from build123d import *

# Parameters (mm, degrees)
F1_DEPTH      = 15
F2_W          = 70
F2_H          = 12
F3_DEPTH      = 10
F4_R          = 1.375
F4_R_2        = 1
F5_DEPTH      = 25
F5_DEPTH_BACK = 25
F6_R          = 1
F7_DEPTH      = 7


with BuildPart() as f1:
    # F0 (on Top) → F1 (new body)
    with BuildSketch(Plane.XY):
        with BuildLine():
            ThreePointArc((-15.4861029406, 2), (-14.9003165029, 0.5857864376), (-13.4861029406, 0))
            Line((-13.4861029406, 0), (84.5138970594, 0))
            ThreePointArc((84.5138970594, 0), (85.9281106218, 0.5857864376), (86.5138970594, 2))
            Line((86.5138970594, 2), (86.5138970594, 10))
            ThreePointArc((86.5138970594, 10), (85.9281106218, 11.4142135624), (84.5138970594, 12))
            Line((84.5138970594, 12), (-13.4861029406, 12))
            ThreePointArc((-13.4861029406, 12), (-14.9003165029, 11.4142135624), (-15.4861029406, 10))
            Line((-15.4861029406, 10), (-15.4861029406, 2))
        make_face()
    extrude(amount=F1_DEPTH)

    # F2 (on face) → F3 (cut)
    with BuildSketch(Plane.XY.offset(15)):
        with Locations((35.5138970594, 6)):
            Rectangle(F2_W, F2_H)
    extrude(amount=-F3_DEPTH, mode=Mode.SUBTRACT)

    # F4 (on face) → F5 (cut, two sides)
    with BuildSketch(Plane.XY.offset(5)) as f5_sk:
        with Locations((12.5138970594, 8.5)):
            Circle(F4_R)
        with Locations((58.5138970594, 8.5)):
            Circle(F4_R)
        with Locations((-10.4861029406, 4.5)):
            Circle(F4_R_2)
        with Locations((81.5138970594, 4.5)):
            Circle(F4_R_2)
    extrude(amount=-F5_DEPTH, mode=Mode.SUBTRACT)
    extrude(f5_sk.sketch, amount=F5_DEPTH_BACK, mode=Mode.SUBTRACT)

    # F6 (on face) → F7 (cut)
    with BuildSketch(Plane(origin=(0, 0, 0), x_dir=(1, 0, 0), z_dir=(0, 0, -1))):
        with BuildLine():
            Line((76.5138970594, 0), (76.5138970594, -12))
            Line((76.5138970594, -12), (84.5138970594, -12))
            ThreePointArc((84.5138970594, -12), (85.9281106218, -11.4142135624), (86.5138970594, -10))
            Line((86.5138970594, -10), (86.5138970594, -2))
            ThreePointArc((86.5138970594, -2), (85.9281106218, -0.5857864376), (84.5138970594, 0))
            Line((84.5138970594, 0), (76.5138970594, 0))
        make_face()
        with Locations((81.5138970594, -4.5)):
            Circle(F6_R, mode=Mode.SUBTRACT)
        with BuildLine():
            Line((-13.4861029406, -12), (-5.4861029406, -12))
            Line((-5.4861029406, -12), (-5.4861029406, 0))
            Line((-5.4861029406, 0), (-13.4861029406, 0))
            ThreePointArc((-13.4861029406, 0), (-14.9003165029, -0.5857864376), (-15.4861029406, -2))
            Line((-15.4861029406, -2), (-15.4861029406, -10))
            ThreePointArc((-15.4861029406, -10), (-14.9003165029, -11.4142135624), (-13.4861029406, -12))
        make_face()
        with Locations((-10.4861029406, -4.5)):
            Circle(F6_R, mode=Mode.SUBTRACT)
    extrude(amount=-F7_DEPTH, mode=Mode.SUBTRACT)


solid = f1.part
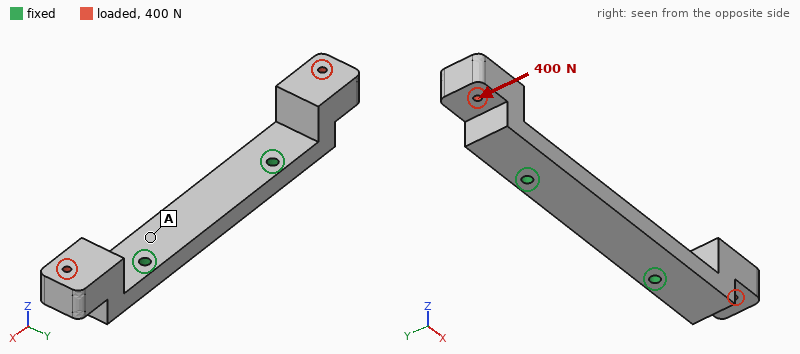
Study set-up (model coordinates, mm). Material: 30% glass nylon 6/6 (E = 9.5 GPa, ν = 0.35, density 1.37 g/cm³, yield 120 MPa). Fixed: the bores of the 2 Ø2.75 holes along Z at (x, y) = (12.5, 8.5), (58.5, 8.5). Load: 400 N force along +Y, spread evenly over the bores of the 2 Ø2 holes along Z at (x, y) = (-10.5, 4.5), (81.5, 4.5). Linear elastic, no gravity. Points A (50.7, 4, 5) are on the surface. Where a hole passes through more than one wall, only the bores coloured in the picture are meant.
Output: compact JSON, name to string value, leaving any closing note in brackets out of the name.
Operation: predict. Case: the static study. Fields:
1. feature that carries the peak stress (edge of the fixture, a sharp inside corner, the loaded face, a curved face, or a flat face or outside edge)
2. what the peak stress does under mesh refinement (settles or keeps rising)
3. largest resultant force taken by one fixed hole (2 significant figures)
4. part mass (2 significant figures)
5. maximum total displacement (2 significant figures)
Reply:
{"feature that carries the peak stress": "edge of the fixture", "what the peak stress does under mesh refinement": "keeps rising", "largest resultant force taken by one fixed hole": "380 N", "part mass": "11 g", "maximum total displacement": "0.54 mm"}
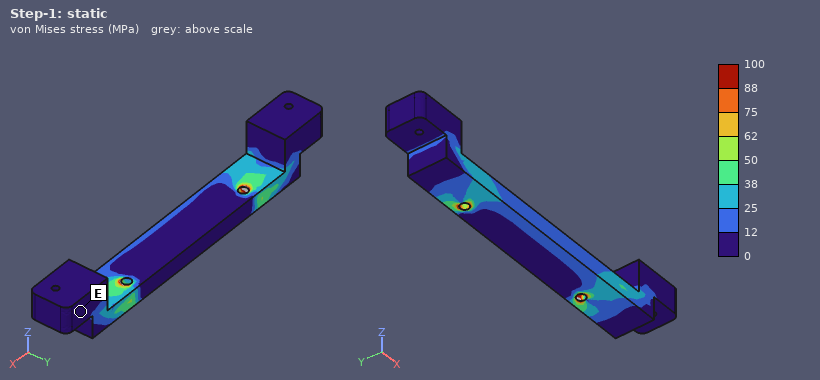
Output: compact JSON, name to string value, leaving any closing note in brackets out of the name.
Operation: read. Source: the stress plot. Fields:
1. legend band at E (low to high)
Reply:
{"legend band at E": "0 to 12 MPa"}
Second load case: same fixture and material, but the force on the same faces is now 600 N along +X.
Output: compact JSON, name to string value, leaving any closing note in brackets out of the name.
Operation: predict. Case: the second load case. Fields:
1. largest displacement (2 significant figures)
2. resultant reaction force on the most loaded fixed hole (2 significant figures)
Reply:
{"largest displacement": "0.84 mm", "resultant reaction force on the most loaded fixed hole": "300 N"}
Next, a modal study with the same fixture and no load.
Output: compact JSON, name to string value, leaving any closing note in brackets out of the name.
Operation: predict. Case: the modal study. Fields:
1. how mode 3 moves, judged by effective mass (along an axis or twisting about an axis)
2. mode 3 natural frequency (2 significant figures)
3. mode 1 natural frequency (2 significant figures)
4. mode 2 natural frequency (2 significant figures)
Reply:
{"how mode 3 moves, judged by effective mass": "along Y", "mode 3 natural frequency": "2600 Hz", "mode 1 natural frequency": "1700 Hz", "mode 2 natural frequency": "1700 Hz"}
